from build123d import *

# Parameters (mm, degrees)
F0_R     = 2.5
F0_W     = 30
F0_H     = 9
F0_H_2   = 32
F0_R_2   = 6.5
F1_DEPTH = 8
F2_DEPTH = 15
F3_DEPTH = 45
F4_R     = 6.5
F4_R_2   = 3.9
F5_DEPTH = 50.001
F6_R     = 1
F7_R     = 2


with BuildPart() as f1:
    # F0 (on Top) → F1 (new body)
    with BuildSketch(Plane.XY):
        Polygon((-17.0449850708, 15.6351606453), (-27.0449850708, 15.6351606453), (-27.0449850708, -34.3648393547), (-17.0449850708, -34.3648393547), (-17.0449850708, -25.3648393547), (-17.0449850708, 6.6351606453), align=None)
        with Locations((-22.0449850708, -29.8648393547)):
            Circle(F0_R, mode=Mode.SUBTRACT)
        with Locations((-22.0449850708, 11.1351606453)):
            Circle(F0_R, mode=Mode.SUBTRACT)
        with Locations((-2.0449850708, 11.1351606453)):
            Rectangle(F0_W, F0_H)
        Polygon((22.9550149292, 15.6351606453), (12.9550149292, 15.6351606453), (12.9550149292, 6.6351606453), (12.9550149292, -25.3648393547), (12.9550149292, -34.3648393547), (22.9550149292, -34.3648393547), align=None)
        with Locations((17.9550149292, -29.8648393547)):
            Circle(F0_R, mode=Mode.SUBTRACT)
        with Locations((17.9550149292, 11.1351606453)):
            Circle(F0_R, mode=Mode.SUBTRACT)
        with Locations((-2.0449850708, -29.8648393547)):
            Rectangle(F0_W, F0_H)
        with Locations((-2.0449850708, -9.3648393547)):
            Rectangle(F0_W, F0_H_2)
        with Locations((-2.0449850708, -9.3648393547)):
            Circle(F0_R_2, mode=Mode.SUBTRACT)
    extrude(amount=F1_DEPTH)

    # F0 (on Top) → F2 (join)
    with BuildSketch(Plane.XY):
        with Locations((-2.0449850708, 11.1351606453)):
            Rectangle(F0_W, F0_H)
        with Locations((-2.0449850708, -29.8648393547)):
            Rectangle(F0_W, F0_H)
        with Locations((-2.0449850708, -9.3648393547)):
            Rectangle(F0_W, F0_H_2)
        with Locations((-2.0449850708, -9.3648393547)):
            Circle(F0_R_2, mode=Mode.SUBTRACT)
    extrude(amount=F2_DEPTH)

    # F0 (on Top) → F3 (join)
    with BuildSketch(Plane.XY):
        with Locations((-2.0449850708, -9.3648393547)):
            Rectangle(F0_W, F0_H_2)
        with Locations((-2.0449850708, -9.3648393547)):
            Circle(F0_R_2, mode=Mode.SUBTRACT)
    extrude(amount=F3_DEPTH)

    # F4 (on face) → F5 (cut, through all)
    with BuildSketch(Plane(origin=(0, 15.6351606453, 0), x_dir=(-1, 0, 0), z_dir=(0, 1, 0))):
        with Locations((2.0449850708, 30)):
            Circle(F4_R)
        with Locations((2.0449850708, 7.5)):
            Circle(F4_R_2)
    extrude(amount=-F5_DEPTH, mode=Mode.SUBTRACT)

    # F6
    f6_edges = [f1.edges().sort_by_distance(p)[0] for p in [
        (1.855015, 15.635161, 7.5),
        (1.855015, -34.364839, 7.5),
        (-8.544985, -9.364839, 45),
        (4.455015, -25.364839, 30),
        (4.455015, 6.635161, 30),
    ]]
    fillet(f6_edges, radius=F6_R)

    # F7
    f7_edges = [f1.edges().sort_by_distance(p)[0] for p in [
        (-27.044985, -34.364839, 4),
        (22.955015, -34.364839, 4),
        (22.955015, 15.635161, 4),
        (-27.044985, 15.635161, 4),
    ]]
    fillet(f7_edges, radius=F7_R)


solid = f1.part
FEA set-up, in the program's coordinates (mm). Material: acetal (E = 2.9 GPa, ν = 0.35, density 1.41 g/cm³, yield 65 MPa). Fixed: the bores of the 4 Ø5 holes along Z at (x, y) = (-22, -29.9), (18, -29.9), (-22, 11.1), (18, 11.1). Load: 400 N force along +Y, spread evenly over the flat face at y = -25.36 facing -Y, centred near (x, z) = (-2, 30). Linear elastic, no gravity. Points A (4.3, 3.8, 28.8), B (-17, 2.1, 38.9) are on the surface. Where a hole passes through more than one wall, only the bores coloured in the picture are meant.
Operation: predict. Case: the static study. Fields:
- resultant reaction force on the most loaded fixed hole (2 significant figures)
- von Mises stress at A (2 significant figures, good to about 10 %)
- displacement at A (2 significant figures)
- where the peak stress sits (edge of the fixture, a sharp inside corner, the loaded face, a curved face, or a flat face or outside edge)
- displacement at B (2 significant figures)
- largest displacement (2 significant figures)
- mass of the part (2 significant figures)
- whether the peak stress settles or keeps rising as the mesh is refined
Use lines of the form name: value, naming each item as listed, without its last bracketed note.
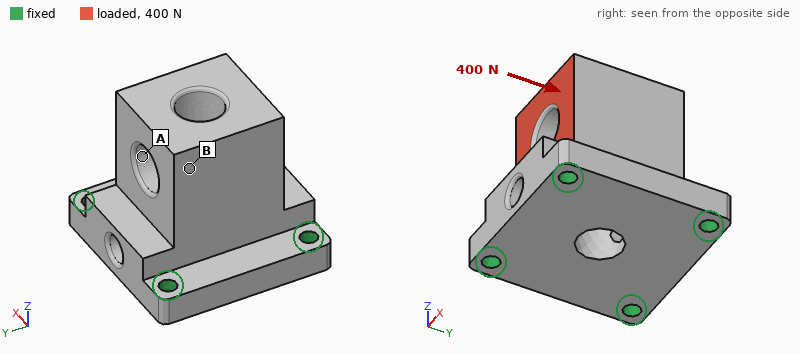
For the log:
resultant reaction force on the most loaded fixed hole: 180 N
von Mises stress at A: 1.2 MPa
displacement at A: 36 µm
where the peak stress sits: edge of the fixture
displacement at B: 50 µm
largest displacement: 65 µm
mass of the part: 68 g
whether the peak stress settles or keeps rising as the mesh is refined: keeps rising
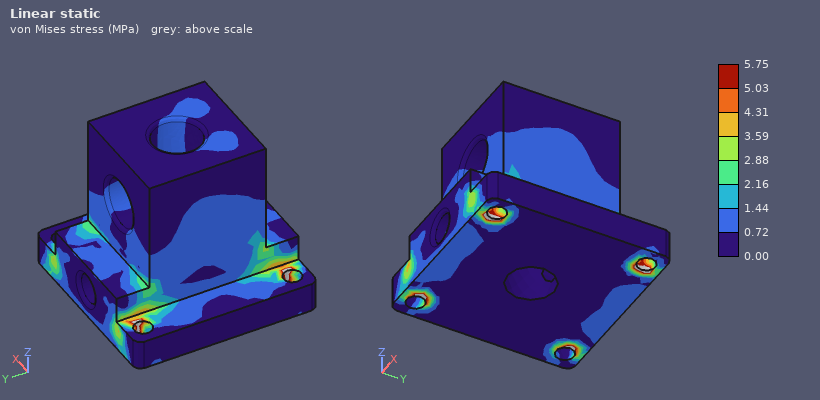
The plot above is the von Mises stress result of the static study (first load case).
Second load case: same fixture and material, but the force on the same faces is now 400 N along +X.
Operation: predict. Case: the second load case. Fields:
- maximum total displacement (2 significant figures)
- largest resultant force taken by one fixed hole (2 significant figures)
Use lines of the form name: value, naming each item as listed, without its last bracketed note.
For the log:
maximum total displacement: 0.11 mm
largest resultant force taken by one fixed hole: 220 N
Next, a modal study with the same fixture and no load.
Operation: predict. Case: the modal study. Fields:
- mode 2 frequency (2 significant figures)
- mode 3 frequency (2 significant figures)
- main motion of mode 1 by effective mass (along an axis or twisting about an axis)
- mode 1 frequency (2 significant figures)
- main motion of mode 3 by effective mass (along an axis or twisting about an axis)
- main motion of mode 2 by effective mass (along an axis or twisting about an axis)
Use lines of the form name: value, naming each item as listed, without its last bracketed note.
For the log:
mode 2 frequency: 2600 Hz
mode 3 frequency: 3600 Hz
main motion of mode 1 by effective mass: along X
mode 1 frequency: 2300 Hz
main motion of mode 3 by effective mass: along Z
main motion of mode 2 by effective mass: along Y
